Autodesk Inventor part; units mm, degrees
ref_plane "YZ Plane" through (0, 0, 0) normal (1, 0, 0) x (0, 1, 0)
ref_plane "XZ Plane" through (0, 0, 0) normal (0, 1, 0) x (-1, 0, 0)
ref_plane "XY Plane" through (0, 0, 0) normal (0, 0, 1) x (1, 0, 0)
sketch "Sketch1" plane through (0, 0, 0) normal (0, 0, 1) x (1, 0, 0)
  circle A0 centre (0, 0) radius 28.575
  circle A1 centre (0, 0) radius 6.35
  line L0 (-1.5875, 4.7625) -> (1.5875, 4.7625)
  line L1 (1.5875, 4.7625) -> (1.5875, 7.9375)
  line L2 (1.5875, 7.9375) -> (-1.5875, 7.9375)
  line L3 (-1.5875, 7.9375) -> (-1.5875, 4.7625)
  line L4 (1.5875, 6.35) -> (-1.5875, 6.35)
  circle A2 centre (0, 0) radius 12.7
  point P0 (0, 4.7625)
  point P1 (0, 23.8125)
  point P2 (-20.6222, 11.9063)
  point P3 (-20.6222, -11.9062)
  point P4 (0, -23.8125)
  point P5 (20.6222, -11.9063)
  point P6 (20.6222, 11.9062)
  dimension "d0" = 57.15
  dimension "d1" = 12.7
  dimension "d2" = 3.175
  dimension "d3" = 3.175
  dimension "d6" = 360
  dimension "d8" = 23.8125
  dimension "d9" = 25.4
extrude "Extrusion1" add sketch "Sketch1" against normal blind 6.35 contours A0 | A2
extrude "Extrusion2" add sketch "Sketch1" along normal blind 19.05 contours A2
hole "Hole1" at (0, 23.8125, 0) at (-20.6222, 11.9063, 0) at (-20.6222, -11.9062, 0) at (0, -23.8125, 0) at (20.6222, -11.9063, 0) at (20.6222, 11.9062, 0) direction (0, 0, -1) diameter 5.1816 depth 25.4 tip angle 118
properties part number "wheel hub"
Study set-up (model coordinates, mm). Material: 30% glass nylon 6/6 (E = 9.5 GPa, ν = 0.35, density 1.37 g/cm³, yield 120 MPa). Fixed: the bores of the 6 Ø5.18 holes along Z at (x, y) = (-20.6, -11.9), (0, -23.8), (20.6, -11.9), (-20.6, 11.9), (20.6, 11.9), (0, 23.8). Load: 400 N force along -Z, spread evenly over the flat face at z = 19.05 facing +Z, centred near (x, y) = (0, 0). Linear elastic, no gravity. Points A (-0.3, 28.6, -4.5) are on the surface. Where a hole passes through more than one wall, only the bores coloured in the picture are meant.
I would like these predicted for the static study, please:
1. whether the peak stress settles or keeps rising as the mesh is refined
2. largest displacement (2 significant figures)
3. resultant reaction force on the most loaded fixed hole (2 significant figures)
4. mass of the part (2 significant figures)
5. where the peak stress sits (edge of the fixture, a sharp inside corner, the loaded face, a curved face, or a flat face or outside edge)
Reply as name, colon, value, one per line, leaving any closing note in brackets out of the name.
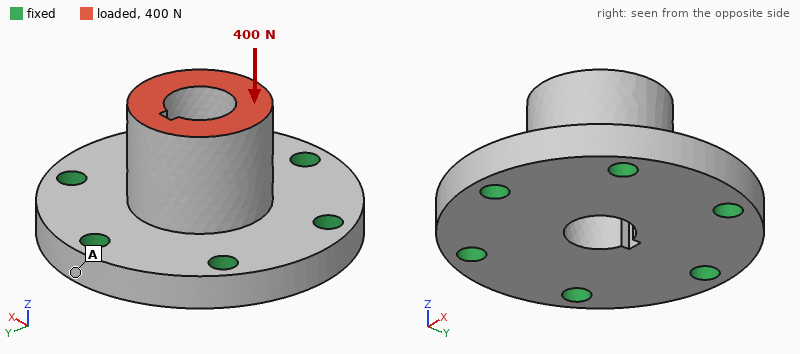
whether the peak stress settles or keeps rising as the mesh is refined: keeps rising
largest displacement: 9.2 µm
resultant reaction force on the most loaded fixed hole: 73 N
mass of the part: 30 g
where the peak stress sits: edge of the fixture
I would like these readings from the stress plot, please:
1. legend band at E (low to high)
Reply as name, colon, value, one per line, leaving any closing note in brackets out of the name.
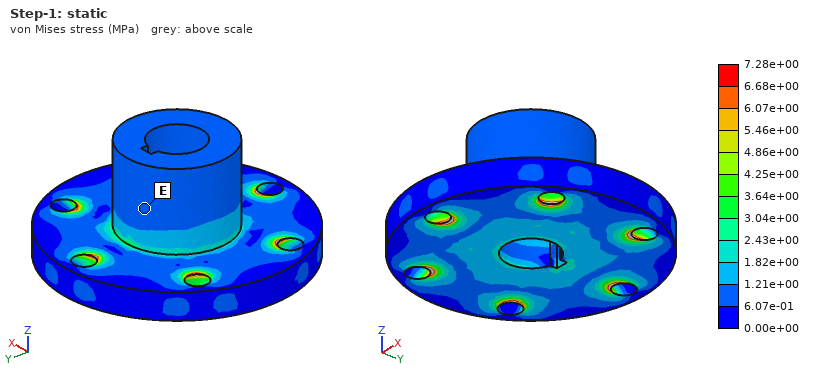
legend band at E: 6.07e-01 to 1.21e+00 MPa
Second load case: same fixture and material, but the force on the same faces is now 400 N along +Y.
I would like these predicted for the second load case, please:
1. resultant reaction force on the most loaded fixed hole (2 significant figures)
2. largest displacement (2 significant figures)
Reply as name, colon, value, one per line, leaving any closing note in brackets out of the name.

resultant reaction force on the most loaded fixed hole: 190 N
largest displacement: 41 µm
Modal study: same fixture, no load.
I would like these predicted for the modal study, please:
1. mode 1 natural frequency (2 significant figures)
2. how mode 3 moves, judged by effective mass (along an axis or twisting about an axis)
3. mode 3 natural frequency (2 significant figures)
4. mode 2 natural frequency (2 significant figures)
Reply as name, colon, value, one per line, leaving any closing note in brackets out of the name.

mode 1 natural frequency: 8200 Hz
how mode 3 moves, judged by effective mass: along Z
mode 3 natural frequency: 9400 Hz
mode 2 natural frequency: 8200 Hz
